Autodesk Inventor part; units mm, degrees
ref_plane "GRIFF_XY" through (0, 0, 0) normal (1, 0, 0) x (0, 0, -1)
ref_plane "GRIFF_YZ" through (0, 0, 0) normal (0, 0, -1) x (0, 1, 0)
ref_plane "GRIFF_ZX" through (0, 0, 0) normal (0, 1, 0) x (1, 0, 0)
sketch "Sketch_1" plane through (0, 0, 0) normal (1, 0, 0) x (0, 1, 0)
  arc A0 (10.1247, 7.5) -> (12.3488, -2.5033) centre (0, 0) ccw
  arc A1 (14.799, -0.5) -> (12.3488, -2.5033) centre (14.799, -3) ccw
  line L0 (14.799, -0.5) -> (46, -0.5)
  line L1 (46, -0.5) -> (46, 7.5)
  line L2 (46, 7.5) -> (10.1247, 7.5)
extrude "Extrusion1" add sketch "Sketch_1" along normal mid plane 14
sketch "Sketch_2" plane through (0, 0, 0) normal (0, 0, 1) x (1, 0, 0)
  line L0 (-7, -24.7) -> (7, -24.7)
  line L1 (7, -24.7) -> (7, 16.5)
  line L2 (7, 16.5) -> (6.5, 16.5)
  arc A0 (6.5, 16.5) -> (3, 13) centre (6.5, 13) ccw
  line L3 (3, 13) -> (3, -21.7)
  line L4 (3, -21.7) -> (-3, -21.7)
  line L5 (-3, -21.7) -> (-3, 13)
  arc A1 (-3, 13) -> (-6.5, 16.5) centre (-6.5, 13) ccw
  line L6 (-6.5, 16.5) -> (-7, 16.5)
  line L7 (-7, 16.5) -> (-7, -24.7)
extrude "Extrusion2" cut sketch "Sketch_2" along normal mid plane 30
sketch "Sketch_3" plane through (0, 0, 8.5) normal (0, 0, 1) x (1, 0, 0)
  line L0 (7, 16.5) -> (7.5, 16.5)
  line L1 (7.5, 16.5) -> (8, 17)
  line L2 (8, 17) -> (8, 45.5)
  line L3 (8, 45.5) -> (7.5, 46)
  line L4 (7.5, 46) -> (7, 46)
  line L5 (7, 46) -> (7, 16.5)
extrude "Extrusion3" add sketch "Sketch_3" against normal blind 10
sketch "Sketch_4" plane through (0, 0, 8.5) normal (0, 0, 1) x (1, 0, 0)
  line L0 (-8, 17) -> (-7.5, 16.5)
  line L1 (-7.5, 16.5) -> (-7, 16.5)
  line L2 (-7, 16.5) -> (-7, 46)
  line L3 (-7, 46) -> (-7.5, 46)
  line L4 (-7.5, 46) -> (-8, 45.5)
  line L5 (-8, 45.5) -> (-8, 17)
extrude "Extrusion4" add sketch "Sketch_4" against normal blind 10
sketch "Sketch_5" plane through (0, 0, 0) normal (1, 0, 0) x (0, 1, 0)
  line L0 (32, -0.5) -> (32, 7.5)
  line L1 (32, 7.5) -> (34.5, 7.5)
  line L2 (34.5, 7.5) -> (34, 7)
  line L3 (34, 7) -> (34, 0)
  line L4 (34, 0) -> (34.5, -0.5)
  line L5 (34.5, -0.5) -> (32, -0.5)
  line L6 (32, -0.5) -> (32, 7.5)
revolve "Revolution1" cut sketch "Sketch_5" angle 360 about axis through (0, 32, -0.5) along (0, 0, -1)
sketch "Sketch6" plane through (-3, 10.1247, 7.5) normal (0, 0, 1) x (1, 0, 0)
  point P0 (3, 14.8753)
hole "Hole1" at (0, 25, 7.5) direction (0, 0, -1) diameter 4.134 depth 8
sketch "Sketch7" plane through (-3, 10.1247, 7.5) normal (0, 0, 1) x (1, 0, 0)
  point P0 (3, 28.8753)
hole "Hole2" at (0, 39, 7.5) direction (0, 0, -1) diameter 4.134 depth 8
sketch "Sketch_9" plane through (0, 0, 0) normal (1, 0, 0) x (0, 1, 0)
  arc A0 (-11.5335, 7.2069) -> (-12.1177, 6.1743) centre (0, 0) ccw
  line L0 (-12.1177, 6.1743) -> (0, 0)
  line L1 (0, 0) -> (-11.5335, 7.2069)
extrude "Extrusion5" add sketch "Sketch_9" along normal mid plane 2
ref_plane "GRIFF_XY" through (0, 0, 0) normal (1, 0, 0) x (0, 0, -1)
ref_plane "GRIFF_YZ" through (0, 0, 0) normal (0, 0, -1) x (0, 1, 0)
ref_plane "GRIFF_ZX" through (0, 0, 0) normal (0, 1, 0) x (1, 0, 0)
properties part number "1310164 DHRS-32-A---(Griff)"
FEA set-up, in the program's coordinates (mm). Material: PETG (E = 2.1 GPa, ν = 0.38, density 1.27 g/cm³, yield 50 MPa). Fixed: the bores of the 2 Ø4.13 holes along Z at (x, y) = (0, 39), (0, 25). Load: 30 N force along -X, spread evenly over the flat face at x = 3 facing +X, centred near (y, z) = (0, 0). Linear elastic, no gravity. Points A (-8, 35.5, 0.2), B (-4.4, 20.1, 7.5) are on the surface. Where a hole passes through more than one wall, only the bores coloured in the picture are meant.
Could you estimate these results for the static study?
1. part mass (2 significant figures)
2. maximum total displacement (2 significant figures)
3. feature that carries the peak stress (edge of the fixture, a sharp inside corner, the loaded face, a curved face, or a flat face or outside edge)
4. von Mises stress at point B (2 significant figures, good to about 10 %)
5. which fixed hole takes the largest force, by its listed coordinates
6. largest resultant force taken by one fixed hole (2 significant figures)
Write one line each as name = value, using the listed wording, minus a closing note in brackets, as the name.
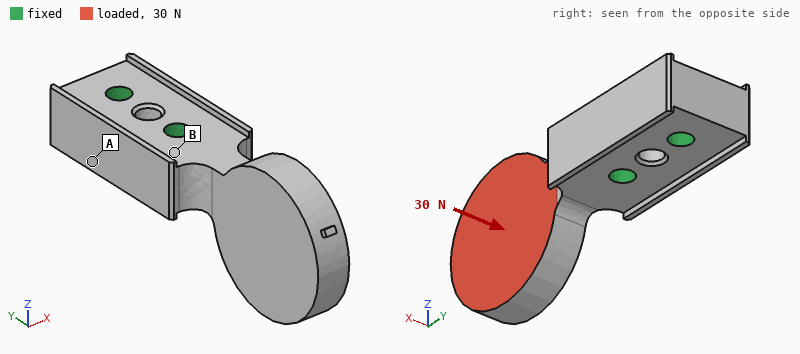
part mass = 8.7 g
maximum total displacement = 0.33 mm
feature that carries the peak stress = a curved face
von Mises stress at point B = 1.8 MPa
which fixed hole takes the largest force, by its listed coordinates = (0, 25)
largest resultant force taken by one fixed hole = 58 N
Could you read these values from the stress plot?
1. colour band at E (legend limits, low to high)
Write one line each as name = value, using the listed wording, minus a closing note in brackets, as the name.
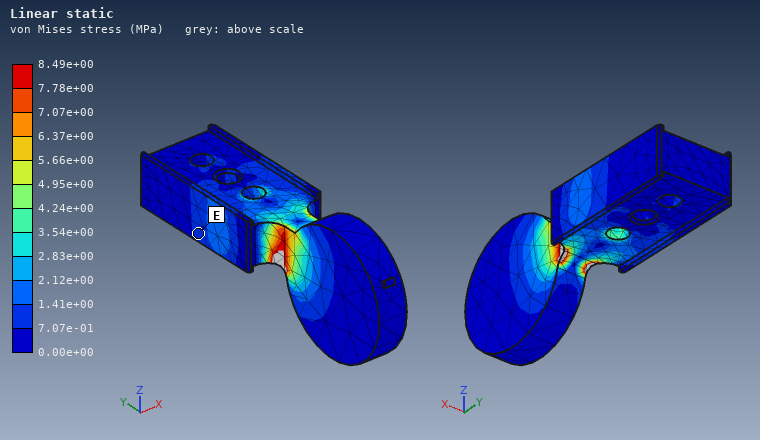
colour band at E = 7.07e-01 to 1.41e+00 MPa
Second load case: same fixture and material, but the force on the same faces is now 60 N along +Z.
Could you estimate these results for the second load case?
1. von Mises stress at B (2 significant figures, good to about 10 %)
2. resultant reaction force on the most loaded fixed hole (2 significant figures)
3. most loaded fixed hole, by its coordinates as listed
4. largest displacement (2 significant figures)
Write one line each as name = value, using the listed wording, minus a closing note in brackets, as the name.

von Mises stress at B = 6.8 MPa
resultant reaction force on the most loaded fixed hole = 83 N
most loaded fixed hole, by its coordinates as listed = (0, 25)
largest displacement = 0.59 mm
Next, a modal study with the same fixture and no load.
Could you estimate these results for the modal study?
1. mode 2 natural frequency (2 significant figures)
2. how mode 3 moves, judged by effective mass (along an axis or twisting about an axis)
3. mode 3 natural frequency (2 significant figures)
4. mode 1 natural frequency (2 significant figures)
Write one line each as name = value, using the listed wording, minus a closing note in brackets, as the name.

mode 2 natural frequency = 970 Hz
how mode 3 moves, judged by effective mass = twisting about Y
mode 3 natural frequency = 2100 Hz
mode 1 natural frequency = 960 Hz
